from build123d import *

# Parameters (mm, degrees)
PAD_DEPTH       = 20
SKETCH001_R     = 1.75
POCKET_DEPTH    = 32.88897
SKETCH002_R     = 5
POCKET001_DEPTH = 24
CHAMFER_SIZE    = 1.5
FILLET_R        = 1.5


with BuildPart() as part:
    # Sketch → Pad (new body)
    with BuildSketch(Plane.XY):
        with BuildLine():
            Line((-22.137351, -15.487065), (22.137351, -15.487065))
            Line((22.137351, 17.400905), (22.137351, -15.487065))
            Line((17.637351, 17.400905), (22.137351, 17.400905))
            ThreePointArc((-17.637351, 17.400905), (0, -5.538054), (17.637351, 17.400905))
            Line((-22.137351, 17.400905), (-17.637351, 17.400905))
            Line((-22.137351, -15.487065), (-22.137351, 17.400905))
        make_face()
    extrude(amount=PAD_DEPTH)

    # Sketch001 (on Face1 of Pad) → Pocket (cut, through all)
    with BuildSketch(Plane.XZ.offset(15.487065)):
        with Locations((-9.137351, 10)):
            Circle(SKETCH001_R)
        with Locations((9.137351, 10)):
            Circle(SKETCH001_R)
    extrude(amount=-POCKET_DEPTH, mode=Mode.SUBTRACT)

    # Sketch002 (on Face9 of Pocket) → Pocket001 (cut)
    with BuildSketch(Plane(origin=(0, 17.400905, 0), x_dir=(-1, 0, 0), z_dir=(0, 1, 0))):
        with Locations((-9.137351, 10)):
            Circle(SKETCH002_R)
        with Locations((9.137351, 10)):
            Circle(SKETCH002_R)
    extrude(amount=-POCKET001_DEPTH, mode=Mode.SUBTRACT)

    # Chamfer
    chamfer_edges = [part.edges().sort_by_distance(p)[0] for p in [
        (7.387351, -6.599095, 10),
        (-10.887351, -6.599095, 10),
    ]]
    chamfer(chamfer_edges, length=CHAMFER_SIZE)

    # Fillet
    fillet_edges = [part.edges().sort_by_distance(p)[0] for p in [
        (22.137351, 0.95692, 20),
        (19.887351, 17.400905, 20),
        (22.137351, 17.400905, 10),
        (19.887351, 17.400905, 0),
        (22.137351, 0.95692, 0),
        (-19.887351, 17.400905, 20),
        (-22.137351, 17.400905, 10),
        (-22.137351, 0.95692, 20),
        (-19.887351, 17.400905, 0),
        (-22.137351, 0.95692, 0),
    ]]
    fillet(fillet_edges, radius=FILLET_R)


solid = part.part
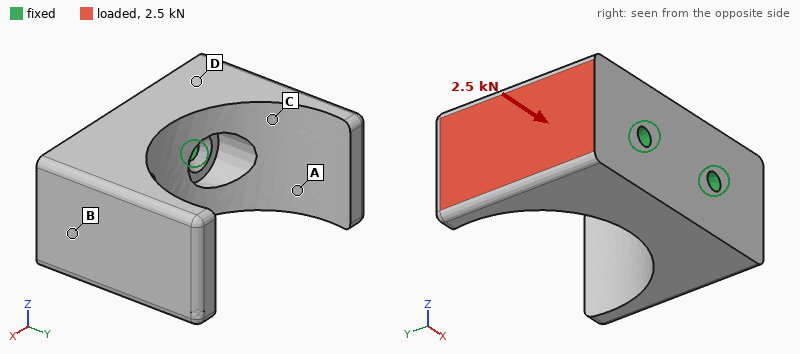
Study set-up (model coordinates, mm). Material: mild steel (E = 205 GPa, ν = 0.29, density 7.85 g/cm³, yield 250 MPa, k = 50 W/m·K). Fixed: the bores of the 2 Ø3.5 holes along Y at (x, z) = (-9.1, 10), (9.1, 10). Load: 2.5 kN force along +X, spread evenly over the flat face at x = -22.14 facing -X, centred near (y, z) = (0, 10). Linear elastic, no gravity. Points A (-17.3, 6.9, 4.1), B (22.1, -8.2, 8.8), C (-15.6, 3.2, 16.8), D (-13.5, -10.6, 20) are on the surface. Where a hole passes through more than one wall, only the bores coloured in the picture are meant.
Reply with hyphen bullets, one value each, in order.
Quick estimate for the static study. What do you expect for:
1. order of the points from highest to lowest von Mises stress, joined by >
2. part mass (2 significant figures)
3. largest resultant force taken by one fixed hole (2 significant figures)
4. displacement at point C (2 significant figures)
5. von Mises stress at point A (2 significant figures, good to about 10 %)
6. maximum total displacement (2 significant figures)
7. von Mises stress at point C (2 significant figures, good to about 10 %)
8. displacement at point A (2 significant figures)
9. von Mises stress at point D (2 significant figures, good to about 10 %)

- C > A > D > B
- 110 g
- 1.7 kN
- 12 µm
- 50 MPa
- 38 µm
- 63 MPa
- 18 µm
- 23 MPa
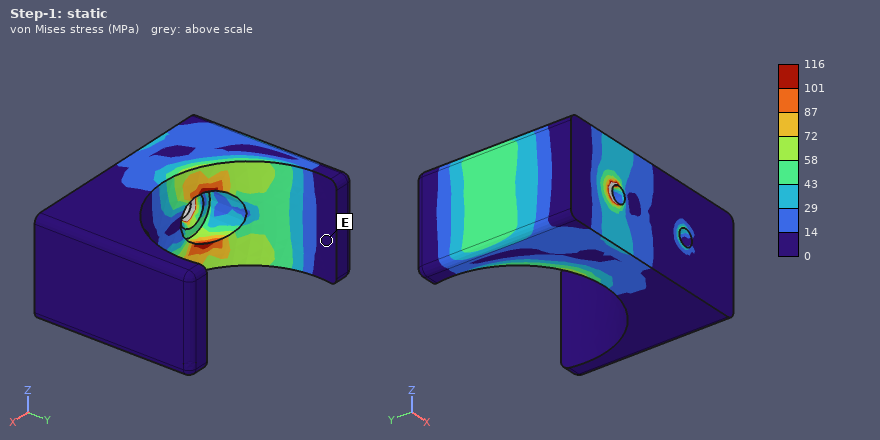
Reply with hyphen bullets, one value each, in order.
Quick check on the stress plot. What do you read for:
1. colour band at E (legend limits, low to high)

- 0 to 14 MPa
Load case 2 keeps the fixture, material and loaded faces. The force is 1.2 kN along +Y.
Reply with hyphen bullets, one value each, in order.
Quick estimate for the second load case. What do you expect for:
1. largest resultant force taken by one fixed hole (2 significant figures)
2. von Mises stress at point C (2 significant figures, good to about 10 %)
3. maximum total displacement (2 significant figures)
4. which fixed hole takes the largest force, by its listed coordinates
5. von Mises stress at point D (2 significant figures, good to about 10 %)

- 1.6 kN
- 10 MPa
- 15 µm
- (-9.1, 10)
- 11 MPa
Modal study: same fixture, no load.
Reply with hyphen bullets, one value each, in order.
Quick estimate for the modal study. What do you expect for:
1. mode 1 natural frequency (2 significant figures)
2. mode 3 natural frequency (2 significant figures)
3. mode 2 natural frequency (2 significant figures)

- 9500 Hz
- 9600 Hz
- 9500 Hz
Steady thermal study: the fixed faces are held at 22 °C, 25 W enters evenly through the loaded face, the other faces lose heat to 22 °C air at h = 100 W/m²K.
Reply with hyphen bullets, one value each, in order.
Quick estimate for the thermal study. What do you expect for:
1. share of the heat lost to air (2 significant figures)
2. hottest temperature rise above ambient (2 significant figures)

- 19 %
- 46 K
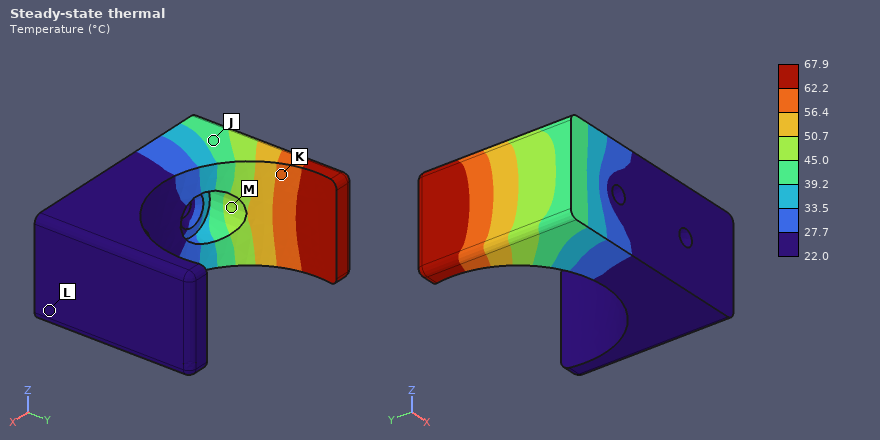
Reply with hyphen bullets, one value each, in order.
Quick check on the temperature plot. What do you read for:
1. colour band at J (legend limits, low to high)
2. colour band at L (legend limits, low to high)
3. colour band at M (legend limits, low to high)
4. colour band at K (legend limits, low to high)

- 39.2 to 45.0 °C
- 22.0 to 27.7 °C
- 45.0 to 50.7 °C
- 56.4 to 62.2 °C
